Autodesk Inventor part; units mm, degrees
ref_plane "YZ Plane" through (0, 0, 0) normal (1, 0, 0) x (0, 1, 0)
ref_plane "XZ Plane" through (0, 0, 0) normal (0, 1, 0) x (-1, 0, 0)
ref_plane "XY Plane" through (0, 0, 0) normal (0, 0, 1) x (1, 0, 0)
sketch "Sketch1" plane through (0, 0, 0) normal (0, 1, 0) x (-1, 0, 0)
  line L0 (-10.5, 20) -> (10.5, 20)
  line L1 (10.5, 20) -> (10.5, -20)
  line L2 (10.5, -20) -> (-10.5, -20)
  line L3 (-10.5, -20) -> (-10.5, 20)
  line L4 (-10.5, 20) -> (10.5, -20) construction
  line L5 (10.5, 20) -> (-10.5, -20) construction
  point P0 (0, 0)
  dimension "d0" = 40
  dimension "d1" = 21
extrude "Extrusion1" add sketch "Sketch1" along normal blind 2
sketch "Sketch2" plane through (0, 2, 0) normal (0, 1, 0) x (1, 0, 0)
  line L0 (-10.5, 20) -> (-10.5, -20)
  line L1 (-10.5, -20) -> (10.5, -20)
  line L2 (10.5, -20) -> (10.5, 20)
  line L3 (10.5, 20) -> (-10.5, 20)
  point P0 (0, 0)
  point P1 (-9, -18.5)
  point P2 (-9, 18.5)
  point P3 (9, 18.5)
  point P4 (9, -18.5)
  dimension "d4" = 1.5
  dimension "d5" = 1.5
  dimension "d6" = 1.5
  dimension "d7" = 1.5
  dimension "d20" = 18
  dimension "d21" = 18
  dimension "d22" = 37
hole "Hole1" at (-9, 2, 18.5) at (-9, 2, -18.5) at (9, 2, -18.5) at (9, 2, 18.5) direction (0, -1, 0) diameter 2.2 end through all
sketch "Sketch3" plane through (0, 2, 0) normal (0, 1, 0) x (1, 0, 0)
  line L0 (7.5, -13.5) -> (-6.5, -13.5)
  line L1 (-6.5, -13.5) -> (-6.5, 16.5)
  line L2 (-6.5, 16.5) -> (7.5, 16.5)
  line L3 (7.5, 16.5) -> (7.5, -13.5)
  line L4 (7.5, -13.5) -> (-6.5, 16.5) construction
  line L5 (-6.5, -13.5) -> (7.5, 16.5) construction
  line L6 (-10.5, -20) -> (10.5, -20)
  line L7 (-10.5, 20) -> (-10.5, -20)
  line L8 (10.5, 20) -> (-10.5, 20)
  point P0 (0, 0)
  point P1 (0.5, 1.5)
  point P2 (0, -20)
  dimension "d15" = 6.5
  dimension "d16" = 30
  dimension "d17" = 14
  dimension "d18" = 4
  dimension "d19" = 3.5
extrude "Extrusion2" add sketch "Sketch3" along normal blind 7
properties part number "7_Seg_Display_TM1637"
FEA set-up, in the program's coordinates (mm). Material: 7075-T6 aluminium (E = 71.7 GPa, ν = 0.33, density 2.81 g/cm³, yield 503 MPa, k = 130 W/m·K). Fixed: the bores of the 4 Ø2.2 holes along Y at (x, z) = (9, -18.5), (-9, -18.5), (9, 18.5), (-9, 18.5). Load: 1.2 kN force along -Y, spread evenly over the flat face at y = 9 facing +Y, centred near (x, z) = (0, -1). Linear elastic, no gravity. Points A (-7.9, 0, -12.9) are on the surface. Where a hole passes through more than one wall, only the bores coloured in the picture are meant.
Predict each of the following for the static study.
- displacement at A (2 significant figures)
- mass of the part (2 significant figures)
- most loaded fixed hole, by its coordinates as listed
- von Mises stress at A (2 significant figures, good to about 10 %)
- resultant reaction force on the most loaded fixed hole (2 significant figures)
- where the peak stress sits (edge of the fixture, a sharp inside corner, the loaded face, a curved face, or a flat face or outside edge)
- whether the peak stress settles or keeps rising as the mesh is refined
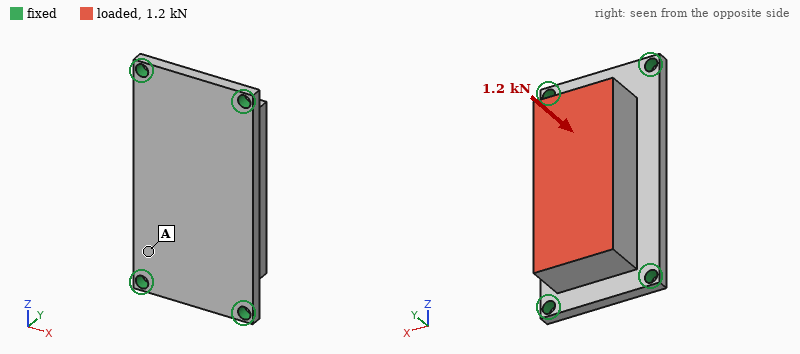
14 µm
13 g
(9, -18.5)
31 MPa
420 N
edge of the fixture
keeps rising
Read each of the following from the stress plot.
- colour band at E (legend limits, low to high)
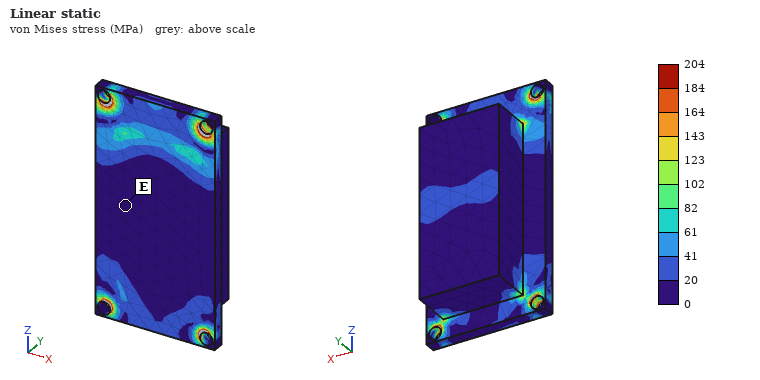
0 to 20 MPa
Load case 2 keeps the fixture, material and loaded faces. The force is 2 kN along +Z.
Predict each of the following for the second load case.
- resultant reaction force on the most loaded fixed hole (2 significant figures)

650 N
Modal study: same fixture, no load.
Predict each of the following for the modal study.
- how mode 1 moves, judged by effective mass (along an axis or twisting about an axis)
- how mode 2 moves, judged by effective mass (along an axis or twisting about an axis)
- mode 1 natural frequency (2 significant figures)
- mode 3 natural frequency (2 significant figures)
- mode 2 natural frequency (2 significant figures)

along Y
along X
10 kHz
20 kHz
14 kHz
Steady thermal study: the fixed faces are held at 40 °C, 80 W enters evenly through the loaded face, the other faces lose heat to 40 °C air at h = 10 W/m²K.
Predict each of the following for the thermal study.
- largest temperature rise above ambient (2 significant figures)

82 K
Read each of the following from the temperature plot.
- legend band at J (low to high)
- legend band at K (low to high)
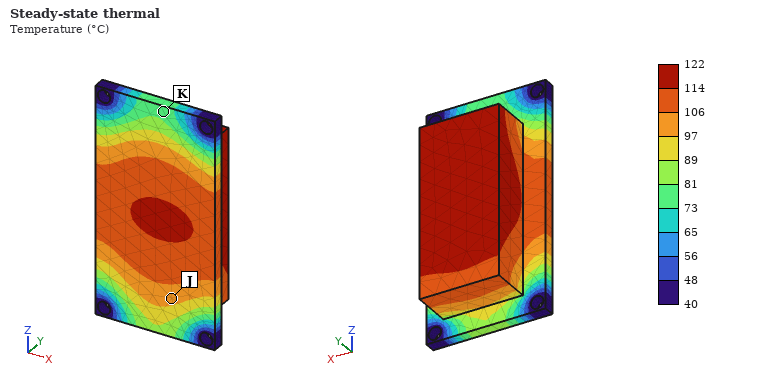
97 to 106 °C
73 to 81 °C
